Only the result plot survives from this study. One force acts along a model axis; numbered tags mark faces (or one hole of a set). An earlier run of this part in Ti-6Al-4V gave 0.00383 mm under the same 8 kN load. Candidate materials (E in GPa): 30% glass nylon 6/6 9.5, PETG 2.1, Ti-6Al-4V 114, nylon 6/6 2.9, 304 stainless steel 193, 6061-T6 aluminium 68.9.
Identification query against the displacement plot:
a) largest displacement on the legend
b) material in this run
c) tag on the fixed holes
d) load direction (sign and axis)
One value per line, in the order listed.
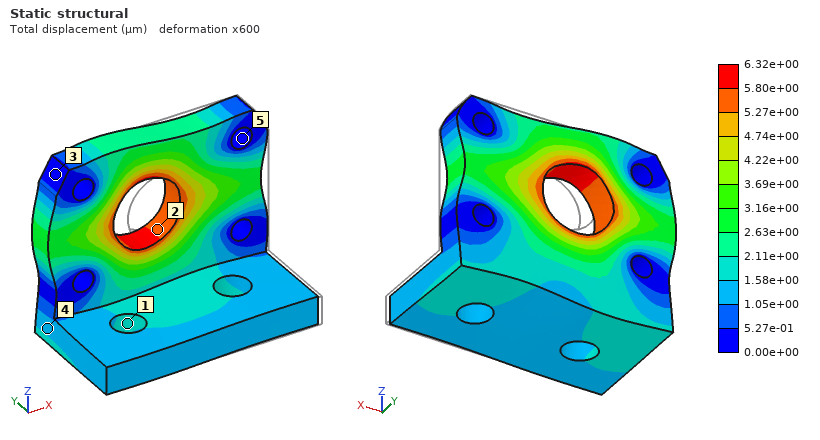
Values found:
6.32e+00 µm
6061-T6 aluminium
5
-X
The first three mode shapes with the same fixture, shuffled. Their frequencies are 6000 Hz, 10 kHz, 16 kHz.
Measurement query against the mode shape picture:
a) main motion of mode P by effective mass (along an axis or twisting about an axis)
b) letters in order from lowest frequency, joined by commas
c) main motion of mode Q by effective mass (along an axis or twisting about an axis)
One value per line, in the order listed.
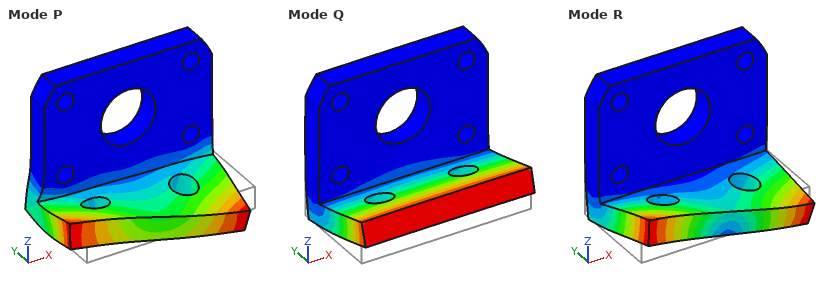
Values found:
along X
Q, R, P
along Z
